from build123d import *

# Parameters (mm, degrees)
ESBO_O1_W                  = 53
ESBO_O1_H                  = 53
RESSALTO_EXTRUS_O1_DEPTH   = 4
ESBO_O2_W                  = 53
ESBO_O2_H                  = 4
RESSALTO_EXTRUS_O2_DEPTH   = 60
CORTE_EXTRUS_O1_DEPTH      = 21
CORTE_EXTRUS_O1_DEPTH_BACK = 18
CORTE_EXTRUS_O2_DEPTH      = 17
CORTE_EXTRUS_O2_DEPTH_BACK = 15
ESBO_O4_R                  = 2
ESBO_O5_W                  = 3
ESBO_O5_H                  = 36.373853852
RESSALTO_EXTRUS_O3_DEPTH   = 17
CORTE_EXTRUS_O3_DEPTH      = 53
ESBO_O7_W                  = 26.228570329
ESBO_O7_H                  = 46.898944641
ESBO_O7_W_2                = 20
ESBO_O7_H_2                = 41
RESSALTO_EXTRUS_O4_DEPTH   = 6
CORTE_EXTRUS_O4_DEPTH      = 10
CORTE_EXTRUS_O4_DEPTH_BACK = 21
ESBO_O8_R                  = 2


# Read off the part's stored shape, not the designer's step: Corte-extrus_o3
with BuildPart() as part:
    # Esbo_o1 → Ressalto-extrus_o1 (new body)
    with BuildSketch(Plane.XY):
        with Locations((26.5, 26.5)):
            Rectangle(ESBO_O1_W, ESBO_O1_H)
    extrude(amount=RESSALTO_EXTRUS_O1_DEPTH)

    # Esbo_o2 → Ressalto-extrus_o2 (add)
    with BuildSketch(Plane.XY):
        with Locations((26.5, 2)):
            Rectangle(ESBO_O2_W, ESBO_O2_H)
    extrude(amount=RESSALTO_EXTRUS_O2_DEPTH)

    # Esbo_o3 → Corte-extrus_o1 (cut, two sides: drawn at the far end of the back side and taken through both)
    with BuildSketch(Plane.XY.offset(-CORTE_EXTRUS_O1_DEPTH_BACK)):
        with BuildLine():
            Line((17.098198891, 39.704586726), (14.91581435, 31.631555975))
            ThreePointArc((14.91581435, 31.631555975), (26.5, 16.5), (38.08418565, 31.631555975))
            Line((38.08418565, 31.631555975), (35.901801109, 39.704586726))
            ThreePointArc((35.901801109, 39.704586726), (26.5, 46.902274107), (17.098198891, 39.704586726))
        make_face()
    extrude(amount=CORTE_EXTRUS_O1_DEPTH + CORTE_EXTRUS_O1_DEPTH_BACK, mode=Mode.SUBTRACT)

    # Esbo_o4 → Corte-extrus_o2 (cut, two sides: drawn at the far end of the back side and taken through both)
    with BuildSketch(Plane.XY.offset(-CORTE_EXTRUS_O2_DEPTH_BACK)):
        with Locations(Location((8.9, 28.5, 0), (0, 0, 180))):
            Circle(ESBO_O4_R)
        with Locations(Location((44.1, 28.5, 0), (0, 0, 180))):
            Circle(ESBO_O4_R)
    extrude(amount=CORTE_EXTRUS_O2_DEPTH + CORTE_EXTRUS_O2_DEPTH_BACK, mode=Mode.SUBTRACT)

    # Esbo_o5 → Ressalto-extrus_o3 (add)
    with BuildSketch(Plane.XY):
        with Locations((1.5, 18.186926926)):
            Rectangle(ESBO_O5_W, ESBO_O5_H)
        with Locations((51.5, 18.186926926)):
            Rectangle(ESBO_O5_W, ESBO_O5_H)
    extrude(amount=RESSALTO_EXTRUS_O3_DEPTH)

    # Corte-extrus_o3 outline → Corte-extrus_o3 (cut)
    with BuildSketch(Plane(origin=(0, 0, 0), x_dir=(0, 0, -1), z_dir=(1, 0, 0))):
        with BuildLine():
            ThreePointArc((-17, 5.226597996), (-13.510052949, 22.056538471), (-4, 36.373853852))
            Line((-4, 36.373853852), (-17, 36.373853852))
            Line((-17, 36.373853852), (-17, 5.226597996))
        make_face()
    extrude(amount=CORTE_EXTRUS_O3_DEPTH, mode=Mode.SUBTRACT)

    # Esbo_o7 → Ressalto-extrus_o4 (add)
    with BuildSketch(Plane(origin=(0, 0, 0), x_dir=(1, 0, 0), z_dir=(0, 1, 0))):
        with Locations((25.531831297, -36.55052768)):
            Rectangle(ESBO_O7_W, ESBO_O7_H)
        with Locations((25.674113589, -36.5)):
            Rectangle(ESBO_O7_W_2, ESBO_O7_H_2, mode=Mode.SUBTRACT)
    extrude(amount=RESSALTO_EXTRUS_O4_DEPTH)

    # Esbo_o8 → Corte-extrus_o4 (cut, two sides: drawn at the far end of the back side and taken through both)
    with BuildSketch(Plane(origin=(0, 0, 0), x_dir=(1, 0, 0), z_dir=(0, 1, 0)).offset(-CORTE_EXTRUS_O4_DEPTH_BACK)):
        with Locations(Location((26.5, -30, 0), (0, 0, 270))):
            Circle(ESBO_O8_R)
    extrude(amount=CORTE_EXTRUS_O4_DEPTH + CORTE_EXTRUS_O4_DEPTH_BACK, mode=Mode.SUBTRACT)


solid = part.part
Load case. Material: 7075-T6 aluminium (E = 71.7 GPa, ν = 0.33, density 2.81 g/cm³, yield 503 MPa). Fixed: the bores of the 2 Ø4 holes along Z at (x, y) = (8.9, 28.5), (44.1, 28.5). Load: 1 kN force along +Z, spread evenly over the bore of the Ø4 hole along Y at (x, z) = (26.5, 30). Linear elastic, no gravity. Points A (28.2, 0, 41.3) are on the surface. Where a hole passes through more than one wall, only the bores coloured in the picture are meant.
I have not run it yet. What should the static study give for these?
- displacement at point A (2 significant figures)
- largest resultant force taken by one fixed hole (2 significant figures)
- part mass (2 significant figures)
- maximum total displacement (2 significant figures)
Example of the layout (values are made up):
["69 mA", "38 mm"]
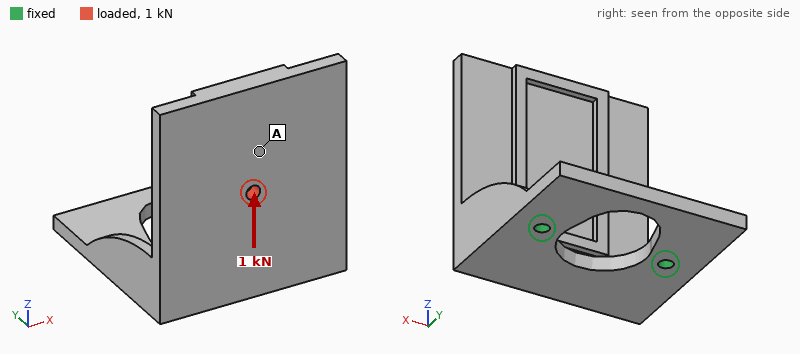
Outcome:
["0.40 mm", "530 N", "65 g", "0.54 mm"]
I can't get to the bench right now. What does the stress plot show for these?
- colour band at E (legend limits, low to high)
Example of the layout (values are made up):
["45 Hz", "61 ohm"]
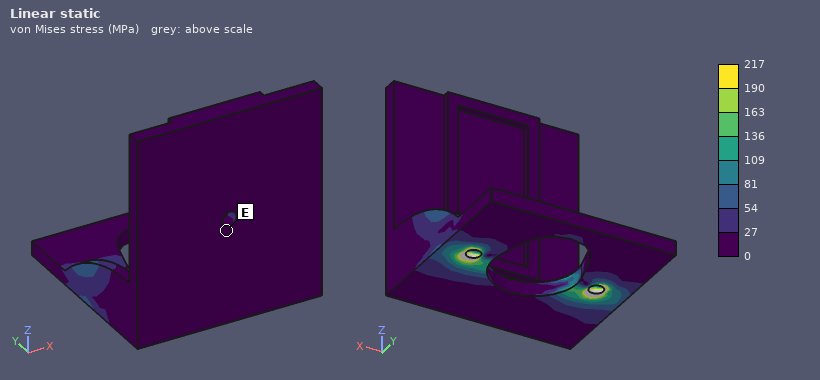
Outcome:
["0 to 27 MPa"]
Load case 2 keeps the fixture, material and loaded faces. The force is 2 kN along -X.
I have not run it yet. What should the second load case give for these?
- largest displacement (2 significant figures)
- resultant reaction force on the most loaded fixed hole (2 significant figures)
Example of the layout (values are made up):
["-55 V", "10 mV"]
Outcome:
["0.90 mm", "2.0 kN"]
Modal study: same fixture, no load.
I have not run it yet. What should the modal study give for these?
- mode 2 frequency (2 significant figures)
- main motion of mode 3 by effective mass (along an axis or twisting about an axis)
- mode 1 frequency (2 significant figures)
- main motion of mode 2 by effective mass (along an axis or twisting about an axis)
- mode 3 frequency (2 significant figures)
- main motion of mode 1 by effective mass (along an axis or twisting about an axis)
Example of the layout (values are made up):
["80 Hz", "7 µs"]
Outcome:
["1400 Hz", "along Z", "840 Hz", "along X", "2300 Hz", "along Y"]
